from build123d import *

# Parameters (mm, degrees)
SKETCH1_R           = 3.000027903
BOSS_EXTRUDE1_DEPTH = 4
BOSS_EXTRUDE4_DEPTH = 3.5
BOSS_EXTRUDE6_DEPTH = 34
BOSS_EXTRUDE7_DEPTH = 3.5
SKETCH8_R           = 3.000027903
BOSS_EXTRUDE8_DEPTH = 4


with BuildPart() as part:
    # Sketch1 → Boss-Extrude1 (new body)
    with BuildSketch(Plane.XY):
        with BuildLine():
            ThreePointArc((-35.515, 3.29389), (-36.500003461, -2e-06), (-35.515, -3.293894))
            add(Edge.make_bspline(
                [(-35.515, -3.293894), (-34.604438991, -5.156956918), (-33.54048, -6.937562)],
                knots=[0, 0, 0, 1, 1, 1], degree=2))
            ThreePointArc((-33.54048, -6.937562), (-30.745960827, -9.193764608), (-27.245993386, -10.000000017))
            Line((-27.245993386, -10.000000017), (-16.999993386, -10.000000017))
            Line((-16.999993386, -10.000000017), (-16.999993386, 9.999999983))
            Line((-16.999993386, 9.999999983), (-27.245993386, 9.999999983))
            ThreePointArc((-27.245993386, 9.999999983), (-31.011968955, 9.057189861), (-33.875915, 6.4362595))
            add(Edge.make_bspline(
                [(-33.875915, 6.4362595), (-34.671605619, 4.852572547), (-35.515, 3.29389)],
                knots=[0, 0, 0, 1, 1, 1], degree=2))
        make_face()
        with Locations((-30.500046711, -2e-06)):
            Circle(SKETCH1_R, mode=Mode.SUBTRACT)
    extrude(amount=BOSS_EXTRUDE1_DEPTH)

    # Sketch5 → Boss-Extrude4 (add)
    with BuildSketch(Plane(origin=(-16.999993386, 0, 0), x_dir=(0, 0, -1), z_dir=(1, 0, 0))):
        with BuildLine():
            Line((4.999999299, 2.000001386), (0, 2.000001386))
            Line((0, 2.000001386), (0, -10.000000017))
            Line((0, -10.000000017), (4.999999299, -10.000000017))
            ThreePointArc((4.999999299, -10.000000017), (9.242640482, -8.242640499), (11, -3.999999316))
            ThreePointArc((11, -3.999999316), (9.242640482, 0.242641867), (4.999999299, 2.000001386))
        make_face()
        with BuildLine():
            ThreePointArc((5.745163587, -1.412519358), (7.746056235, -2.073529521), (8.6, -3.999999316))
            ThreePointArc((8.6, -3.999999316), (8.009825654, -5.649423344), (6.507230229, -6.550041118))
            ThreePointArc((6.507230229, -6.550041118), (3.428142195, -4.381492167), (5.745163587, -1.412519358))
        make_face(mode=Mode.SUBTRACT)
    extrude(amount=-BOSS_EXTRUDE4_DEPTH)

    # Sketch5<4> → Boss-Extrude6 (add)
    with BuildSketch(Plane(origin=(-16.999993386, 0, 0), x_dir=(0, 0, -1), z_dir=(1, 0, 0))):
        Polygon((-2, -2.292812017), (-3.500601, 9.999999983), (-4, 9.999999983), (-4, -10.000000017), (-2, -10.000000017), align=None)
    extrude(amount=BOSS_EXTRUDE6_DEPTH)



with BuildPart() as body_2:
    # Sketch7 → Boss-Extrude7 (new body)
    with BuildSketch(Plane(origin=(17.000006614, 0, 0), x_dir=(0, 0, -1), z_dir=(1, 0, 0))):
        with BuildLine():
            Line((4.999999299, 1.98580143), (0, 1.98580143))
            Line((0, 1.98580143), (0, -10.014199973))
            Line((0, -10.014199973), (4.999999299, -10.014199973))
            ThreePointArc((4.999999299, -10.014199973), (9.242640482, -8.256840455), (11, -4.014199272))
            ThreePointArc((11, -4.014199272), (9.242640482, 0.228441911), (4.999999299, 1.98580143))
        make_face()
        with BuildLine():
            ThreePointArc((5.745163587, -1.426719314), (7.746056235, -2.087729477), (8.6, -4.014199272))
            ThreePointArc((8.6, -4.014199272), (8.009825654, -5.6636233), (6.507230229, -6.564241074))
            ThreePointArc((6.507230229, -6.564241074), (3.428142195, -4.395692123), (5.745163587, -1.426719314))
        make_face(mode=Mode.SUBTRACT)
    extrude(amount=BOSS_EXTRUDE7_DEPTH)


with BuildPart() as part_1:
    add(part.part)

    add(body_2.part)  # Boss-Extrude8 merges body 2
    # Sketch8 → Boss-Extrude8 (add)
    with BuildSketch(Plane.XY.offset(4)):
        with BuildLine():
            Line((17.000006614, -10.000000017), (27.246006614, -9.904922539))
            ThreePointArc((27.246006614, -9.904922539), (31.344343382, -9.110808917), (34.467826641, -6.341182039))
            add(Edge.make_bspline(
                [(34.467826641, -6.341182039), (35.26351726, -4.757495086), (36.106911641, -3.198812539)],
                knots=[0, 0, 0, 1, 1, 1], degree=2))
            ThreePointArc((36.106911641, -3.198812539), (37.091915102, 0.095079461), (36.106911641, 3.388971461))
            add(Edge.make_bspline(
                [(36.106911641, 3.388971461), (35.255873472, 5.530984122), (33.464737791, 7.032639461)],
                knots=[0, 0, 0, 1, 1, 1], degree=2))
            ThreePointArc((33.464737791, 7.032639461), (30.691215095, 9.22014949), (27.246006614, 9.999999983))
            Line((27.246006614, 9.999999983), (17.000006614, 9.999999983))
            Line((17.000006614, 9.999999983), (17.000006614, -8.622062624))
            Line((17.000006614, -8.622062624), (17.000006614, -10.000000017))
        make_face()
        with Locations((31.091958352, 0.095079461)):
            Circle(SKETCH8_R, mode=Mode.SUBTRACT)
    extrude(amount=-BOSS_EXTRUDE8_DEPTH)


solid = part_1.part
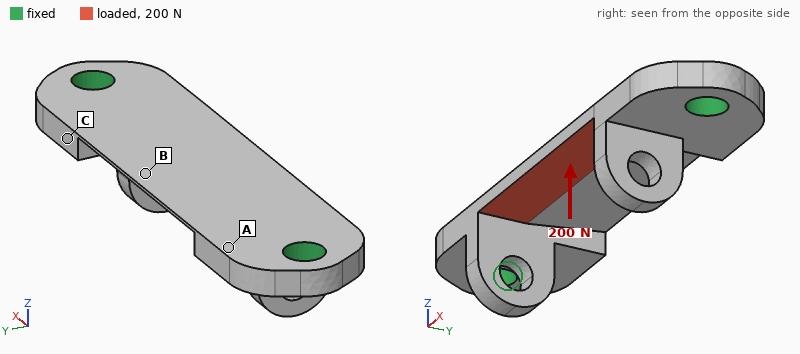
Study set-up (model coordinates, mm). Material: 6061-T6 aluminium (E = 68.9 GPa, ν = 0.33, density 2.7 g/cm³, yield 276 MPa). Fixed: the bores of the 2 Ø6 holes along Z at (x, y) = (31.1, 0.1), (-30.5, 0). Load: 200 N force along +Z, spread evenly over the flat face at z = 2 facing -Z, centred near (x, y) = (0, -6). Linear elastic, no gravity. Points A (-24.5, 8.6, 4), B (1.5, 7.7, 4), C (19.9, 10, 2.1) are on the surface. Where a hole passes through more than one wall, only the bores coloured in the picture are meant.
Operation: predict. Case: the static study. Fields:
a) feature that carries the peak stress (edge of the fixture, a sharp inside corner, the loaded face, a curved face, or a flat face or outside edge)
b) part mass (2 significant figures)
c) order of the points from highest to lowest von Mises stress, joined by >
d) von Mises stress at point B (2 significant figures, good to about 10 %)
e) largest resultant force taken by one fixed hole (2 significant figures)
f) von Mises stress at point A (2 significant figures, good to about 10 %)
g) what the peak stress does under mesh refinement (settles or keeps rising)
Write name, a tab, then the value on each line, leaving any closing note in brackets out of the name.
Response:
feature that carries the peak stress	edge of the fixture
part mass	12 g
order of the points from highest to lowest von Mises stress, joined by >	B > A > C
von Mises stress at point B	22 MPa
largest resultant force taken by one fixed hole	190 N
von Mises stress at point A	12 MPa
what the peak stress does under mesh refinement	keeps rising
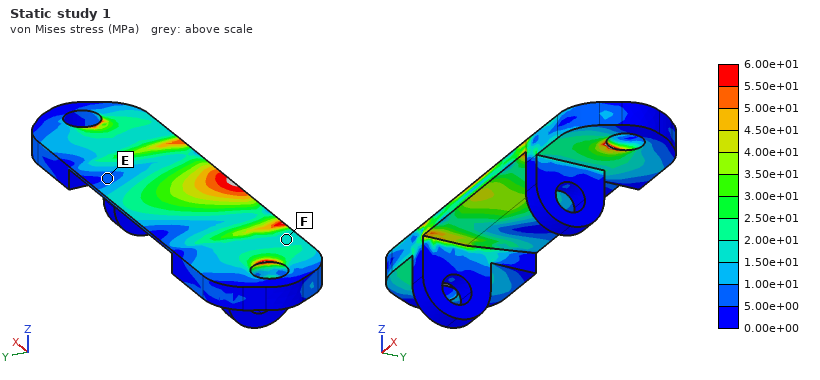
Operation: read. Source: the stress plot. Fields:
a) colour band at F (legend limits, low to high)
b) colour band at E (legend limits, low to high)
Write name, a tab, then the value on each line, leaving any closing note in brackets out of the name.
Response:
colour band at F	1.50e+01 to 2.00e+01 MPa
colour band at E	5.00e+00 to 1.00e+01 MPa
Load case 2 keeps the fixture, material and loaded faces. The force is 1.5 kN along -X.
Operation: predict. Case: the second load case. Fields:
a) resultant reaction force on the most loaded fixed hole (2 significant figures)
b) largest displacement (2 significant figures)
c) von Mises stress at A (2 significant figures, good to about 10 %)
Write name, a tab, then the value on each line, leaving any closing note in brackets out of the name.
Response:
resultant reaction force on the most loaded fixed hole	770 N
largest displacement	21 µm
von Mises stress at A	13 MPa
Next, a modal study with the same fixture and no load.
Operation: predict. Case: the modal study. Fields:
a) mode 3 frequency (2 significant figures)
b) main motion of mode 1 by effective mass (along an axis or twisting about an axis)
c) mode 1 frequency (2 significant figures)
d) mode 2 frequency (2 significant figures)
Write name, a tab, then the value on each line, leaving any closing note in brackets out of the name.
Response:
mode 3 frequency	9500 Hz
main motion of mode 1 by effective mass	along Z
mode 1 frequency	5300 Hz
mode 2 frequency	8600 Hz
